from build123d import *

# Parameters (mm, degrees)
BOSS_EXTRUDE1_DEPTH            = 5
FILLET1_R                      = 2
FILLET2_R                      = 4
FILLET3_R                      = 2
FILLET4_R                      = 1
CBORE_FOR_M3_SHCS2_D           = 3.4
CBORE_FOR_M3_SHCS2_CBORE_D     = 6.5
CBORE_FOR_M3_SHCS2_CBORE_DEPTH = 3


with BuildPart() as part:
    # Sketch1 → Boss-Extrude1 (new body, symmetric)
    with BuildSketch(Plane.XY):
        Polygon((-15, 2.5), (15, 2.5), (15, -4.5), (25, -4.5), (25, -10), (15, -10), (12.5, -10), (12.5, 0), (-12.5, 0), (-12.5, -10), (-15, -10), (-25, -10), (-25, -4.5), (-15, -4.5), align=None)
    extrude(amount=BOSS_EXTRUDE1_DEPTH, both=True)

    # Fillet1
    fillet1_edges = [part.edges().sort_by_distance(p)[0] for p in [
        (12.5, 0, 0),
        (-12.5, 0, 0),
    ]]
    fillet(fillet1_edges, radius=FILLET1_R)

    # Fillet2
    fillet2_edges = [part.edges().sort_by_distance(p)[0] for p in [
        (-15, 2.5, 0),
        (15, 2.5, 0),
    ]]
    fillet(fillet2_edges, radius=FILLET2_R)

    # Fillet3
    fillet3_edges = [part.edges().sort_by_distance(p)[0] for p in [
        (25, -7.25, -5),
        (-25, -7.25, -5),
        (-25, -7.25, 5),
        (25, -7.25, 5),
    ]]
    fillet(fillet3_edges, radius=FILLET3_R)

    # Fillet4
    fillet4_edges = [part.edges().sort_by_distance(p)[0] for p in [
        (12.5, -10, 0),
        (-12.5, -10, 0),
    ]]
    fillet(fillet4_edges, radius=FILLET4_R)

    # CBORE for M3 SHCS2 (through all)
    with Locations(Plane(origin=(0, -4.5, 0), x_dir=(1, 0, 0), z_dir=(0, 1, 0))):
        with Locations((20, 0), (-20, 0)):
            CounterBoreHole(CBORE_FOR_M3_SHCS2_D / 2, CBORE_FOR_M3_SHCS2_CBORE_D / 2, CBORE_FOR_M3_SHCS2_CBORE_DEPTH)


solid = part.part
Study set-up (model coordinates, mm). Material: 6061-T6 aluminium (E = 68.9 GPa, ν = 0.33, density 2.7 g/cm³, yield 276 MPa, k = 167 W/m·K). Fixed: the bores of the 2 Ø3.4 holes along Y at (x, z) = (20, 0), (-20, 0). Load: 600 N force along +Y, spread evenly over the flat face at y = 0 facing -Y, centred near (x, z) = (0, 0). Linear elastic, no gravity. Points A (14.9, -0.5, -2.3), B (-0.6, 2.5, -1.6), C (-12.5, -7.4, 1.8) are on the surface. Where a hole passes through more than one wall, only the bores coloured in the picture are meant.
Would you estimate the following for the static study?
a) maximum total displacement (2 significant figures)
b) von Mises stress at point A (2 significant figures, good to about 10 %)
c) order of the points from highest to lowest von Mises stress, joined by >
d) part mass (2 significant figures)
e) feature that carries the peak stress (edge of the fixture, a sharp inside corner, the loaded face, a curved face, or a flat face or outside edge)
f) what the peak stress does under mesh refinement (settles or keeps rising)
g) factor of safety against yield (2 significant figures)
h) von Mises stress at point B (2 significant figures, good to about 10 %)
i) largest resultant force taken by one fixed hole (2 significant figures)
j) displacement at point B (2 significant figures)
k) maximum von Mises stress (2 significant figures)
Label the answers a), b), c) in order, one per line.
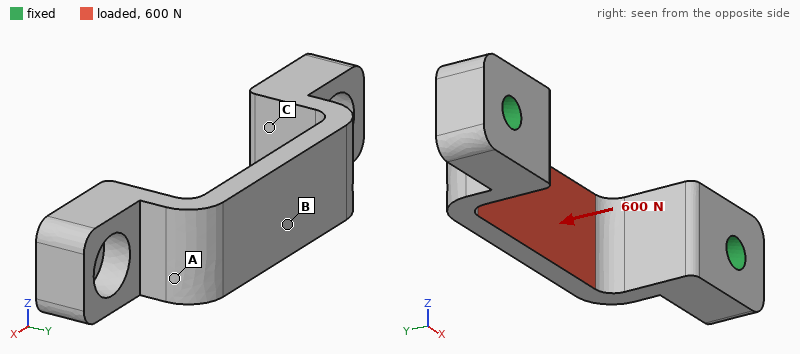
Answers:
a) 56 µm
b) 45 MPa
c) B > A > C
d) 5.5 g
e) a curved face
f) settles
g) 2.0
h) 95 MPa
i) 430 N
j) 53 µm
k) 140 MPa
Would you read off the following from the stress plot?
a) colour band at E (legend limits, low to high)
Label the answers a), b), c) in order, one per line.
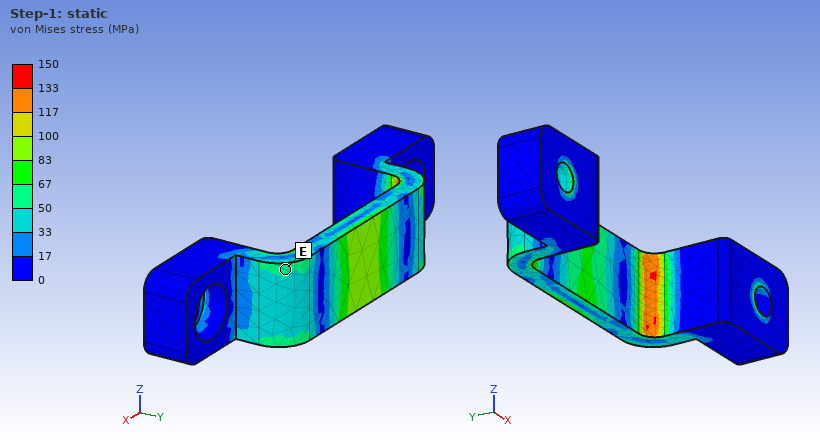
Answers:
a) 50 to 67 MPa
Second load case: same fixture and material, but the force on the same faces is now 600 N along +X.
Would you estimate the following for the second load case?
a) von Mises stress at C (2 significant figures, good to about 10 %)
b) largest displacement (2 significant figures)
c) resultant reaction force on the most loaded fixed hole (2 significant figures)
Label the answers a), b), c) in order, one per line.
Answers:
a) 21 MPa
b) 44 µm
c) 300 N
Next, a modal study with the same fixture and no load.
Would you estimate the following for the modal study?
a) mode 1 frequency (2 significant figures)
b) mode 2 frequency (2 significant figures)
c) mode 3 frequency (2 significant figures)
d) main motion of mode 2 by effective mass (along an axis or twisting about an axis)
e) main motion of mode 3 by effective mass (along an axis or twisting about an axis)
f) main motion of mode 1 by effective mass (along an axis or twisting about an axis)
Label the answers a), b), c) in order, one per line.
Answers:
a) 11 kHz
b) 13 kHz
c) 16 kHz
d) along X
e) along Y
f) along Z
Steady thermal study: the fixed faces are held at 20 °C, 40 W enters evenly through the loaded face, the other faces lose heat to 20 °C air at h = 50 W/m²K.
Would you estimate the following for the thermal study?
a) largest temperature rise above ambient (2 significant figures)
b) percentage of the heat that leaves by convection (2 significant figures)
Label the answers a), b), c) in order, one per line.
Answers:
a) 82 K
b) 5.9 %
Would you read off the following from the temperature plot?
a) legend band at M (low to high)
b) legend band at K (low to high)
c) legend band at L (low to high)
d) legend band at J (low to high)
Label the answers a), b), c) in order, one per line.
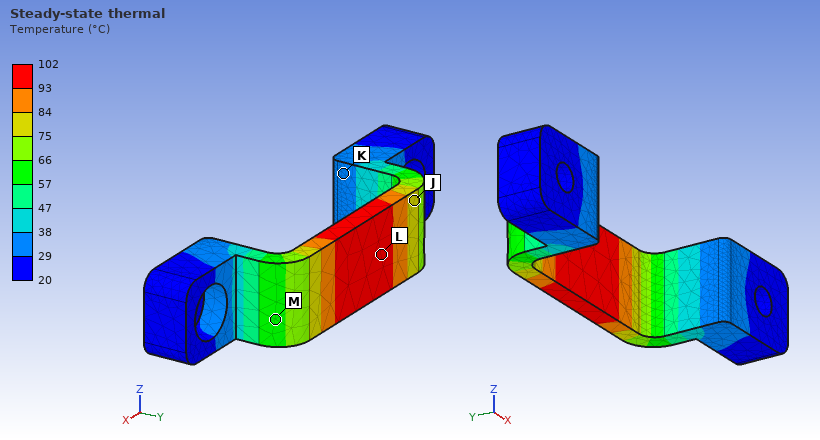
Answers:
a) 57 to 66 °C
b) 29 to 38 °C
c) 93 to 102 °C
d) 75 to 84 °C
